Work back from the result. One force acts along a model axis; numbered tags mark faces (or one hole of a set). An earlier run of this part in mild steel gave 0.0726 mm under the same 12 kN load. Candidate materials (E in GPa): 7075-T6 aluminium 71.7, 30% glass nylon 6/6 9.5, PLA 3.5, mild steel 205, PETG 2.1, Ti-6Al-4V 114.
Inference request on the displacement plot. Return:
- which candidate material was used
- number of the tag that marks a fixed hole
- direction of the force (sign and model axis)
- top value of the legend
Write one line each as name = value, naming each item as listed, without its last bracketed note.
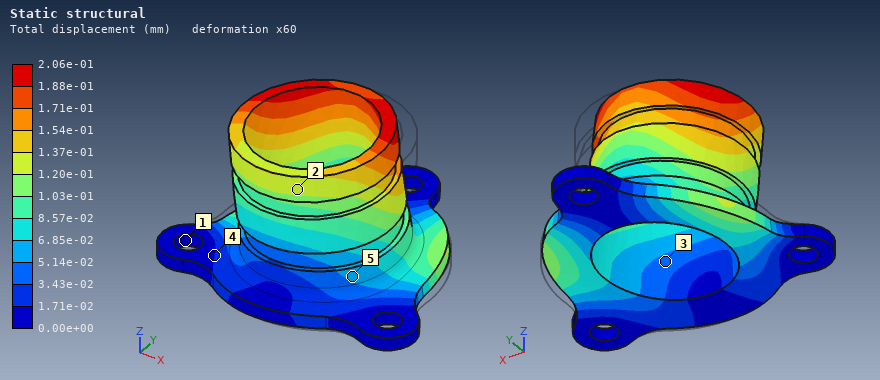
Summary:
which candidate material was used = 7075-T6 aluminium
number of the tag that marks a fixed hole = 1
direction of the force = -X
top value of the legend = 2.06e-01 mm
